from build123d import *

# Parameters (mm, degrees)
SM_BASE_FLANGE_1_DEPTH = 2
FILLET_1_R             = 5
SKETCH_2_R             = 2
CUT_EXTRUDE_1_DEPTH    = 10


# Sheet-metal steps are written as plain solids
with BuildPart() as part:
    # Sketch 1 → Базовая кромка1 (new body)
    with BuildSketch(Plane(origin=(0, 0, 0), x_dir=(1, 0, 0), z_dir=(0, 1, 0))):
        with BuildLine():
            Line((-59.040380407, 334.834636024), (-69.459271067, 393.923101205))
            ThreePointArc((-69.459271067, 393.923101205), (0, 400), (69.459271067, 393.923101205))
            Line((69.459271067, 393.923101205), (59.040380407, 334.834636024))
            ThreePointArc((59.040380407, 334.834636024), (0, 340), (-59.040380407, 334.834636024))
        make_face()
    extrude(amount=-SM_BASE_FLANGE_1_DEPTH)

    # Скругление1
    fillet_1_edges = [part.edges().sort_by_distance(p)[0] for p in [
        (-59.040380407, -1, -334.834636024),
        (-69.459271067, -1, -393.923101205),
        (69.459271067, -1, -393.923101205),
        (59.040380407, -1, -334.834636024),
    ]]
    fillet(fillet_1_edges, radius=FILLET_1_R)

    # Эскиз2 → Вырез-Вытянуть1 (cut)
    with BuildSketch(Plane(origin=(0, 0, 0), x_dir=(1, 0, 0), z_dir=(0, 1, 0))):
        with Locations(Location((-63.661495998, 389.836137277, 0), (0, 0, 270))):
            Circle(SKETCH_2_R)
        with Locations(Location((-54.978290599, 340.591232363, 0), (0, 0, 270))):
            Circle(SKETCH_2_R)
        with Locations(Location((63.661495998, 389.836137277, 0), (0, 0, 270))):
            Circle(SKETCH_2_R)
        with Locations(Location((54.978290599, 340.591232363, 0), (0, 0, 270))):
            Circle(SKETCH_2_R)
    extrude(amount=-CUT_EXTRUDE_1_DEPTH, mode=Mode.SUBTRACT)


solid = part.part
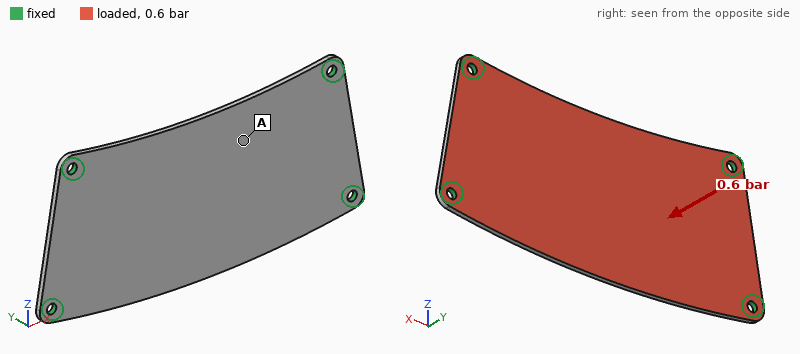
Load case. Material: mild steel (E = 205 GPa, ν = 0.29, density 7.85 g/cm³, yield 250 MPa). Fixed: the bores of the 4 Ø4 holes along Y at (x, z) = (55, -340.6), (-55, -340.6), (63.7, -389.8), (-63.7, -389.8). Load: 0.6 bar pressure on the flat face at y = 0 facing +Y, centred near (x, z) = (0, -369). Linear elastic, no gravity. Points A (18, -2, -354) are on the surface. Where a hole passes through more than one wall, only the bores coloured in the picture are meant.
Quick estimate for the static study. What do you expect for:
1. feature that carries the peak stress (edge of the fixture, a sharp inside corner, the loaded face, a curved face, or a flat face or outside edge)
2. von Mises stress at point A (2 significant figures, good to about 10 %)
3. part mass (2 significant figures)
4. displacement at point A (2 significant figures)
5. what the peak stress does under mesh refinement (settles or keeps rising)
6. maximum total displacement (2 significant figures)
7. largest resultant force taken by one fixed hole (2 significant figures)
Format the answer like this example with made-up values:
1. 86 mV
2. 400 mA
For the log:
1. edge of the fixture
2. 39 MPa
3. 120 g
4. 0.21 mm
5. keeps rising
6. 0.36 mm
7. 120 N
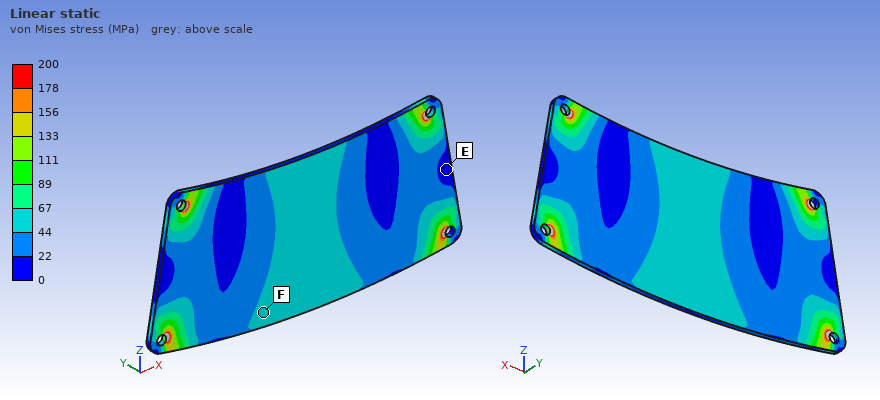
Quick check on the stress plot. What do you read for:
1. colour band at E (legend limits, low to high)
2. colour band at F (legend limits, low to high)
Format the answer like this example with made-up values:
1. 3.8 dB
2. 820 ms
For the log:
1. 0 to 22 MPa
2. 44 to 67 MPa
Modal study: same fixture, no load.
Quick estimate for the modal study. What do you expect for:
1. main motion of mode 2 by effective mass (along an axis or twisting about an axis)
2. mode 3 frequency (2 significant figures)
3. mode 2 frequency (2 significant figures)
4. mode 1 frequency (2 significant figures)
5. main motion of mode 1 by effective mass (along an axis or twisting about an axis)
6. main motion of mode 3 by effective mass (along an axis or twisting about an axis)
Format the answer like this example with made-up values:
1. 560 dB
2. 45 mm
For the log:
1. twisting about X
2. 1800 Hz
3. 1300 Hz
4. 660 Hz
5. along Y
6. twisting about Z
